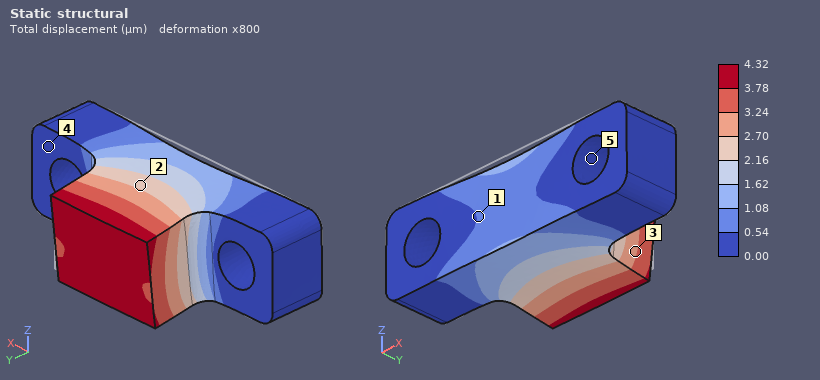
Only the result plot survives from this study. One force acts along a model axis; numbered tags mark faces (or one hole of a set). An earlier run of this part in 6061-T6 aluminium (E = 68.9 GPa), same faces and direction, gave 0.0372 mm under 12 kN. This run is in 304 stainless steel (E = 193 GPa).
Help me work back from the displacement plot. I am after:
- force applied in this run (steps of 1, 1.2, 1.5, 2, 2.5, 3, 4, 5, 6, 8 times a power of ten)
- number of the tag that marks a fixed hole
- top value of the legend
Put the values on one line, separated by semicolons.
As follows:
4 kN; 5; 4.32 µm
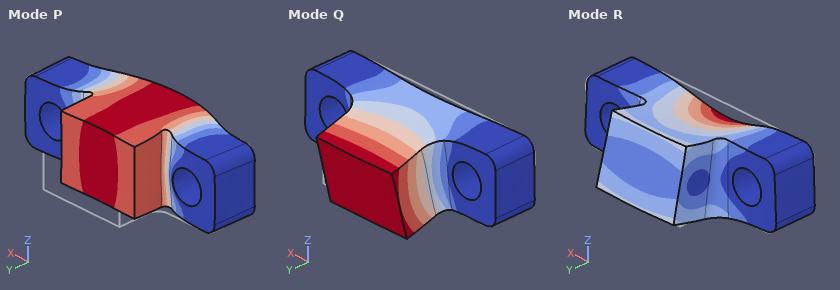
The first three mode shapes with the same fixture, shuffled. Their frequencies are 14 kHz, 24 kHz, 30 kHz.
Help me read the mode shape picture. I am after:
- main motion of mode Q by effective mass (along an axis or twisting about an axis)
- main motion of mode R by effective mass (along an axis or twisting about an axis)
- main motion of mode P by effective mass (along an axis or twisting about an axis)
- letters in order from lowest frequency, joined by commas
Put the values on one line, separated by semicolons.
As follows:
along Z; along Z; along Y; Q, P, R
